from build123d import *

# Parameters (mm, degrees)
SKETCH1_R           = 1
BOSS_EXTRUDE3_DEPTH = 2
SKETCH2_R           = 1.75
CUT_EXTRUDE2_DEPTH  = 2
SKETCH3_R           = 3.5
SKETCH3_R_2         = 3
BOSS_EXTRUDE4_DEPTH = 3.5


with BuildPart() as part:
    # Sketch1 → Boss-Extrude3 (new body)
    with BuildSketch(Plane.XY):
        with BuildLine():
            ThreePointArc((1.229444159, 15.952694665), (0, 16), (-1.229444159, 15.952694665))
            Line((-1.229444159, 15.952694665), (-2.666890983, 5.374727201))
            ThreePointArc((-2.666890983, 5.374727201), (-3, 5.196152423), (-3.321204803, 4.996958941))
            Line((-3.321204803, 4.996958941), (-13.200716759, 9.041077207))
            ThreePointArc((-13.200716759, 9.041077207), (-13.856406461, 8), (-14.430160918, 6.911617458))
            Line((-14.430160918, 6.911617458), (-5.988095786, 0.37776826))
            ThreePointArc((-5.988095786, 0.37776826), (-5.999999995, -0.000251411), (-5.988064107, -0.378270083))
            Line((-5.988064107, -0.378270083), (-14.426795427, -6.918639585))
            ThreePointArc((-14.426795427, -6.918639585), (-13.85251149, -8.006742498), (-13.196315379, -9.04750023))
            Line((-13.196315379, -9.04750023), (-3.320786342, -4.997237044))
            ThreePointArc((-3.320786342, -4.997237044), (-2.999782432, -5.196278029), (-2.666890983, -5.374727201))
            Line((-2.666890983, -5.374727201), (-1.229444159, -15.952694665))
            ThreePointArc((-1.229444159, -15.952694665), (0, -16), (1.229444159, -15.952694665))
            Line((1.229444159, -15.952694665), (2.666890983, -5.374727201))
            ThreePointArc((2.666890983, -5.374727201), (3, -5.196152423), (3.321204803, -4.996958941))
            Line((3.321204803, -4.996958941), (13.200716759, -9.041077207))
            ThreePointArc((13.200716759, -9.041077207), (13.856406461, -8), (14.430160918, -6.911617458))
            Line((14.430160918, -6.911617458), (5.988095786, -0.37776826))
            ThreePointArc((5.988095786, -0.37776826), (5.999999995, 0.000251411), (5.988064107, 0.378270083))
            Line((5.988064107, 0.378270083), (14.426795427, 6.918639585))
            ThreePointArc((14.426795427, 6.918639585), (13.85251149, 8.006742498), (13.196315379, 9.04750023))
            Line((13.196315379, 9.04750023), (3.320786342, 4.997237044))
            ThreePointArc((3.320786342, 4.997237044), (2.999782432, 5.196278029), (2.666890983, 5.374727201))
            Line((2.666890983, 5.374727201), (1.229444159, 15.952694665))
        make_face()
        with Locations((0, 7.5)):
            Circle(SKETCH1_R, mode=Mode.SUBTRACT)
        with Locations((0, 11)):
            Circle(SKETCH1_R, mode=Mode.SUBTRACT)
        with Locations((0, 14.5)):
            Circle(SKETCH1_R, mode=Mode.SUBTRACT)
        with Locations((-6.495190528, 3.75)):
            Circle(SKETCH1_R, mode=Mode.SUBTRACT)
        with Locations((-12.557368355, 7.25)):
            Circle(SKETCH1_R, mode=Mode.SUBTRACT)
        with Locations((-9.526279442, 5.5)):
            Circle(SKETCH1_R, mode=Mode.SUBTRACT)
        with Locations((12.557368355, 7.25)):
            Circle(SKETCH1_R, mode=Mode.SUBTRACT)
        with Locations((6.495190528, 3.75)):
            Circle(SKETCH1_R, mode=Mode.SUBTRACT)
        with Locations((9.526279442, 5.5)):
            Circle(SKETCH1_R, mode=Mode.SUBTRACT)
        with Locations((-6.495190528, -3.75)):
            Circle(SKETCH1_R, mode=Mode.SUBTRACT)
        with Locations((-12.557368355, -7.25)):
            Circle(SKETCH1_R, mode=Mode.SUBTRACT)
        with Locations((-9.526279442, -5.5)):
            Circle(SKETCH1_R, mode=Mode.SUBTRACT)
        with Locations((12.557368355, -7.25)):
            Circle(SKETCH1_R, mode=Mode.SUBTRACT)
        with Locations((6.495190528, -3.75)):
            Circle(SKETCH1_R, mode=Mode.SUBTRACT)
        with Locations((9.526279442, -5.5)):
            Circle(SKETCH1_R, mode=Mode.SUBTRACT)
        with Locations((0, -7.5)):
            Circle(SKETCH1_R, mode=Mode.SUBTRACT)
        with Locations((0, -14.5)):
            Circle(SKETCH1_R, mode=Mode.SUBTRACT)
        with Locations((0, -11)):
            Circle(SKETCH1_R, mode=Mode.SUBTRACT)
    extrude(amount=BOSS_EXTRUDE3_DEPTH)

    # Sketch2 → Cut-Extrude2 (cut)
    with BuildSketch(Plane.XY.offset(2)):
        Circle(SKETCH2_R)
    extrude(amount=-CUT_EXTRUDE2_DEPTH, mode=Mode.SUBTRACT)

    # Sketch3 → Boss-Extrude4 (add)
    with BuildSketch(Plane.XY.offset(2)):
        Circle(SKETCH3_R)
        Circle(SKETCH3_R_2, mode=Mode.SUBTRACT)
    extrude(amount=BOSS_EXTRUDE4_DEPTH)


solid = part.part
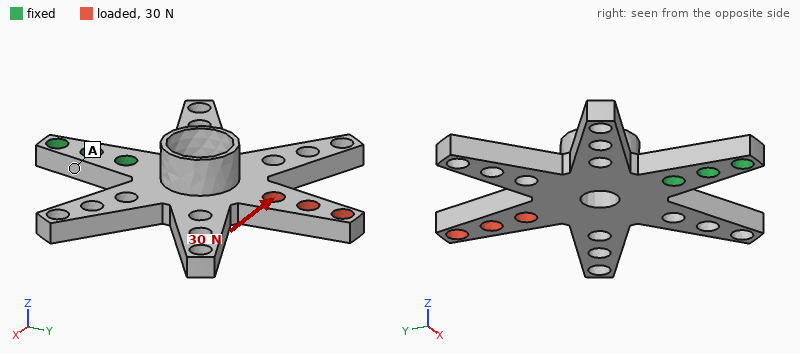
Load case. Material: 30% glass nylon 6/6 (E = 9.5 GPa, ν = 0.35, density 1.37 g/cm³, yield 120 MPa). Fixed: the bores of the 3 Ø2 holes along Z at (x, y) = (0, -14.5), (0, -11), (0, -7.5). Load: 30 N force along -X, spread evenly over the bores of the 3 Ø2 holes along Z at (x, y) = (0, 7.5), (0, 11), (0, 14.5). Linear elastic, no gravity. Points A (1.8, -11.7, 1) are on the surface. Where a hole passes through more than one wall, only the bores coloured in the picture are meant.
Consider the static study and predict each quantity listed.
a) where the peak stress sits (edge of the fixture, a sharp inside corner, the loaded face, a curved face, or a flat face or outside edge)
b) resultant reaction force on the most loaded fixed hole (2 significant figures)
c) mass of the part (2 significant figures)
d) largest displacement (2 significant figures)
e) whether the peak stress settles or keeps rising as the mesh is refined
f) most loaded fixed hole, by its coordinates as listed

edge of the fixture
75 N
0.82 g
0.35 mm
keeps rising
(0, -7.5)
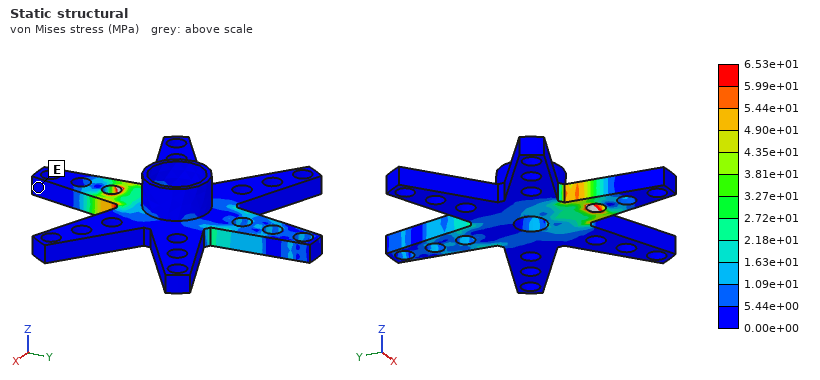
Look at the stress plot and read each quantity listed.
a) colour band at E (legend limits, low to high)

0.00e+00 to 5.44e+00 MPa
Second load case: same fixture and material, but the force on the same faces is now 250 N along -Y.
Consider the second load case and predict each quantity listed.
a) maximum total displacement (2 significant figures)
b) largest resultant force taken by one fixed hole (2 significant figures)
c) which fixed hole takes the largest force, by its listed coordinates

77 µm
230 N
(0, -7.5)
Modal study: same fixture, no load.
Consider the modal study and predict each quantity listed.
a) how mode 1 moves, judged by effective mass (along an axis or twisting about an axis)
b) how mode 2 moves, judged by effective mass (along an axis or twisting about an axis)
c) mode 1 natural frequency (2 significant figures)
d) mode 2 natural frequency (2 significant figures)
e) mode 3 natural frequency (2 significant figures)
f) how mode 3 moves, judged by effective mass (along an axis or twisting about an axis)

along Z
twisting about Y
1900 Hz
2800 Hz
3300 Hz
along X
